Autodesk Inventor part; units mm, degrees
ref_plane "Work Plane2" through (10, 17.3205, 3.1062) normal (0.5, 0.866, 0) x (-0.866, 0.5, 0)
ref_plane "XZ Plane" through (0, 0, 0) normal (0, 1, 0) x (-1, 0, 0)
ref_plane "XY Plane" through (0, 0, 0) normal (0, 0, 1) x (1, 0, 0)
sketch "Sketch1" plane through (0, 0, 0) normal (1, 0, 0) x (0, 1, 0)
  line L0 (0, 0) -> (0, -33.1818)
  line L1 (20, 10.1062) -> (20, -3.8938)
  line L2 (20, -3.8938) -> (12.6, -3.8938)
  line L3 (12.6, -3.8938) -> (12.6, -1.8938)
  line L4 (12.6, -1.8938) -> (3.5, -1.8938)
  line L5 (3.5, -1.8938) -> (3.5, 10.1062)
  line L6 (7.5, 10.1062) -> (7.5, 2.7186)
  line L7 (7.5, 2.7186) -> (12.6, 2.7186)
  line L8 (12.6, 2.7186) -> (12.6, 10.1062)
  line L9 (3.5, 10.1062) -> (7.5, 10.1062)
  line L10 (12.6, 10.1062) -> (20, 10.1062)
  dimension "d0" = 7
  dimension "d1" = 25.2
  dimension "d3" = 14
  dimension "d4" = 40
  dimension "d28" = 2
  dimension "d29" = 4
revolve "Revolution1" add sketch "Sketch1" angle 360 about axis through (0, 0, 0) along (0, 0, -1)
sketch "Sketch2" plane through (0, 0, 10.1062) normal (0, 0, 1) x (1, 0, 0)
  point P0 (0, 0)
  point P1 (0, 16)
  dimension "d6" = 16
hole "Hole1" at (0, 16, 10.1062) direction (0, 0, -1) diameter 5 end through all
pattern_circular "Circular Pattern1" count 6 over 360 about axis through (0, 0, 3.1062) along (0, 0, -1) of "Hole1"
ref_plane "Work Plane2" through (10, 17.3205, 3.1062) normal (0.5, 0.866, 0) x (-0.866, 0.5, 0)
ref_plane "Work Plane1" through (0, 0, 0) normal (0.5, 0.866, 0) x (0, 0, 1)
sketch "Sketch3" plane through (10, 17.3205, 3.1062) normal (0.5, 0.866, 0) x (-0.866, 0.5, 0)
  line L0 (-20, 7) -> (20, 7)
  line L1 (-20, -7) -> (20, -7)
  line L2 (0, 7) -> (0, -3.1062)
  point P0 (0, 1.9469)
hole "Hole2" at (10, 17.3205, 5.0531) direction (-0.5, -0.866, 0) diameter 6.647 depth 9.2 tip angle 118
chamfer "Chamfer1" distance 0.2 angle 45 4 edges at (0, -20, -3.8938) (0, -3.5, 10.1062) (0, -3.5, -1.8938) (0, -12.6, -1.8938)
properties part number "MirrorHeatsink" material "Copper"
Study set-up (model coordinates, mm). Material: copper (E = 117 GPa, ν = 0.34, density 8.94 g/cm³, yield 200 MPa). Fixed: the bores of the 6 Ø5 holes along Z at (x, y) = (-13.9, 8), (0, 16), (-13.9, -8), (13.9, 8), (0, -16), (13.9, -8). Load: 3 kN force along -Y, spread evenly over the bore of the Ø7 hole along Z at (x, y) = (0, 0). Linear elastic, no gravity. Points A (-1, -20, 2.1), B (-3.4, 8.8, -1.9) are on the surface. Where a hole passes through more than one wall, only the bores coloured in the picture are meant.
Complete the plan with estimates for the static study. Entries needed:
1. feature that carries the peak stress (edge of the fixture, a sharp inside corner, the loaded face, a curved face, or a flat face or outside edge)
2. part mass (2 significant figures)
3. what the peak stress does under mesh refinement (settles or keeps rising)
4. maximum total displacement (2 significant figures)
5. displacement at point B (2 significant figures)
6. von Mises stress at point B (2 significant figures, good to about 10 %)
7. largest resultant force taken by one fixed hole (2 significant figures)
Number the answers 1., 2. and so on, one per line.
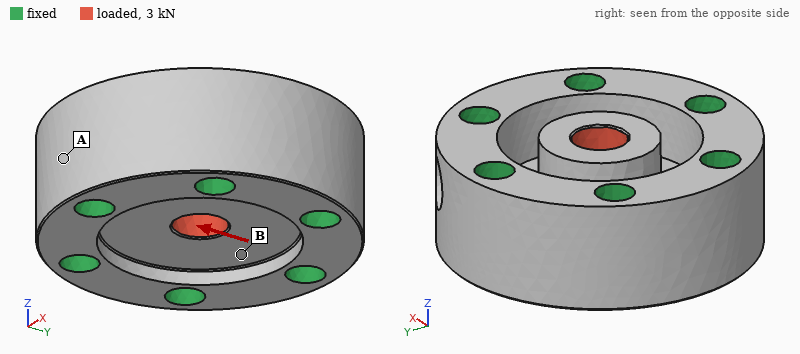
1. a sharp inside corner
2. 110 g
3. keeps rising
4. 5.9 µm
5. 1.3 µm
6. 8.7 MPa
7. 860 N
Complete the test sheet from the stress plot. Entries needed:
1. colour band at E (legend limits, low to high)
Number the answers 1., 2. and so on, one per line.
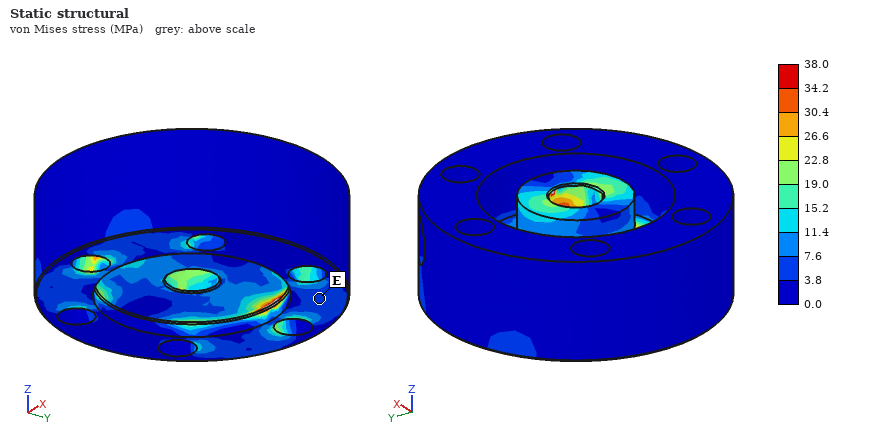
1. 3.8 to 7.6 MPa
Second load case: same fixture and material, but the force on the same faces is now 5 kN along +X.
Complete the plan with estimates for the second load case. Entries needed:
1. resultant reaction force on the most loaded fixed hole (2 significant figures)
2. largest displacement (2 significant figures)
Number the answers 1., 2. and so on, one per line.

1. 1.3 kN
2. 9.8 µm
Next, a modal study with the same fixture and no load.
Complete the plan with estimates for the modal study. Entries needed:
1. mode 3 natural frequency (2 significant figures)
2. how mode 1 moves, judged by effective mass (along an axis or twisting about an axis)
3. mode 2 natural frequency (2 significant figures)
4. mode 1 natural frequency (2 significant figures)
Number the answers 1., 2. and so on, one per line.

1. 33 kHz
2. along Z
3. 33 kHz
4. 31 kHz
